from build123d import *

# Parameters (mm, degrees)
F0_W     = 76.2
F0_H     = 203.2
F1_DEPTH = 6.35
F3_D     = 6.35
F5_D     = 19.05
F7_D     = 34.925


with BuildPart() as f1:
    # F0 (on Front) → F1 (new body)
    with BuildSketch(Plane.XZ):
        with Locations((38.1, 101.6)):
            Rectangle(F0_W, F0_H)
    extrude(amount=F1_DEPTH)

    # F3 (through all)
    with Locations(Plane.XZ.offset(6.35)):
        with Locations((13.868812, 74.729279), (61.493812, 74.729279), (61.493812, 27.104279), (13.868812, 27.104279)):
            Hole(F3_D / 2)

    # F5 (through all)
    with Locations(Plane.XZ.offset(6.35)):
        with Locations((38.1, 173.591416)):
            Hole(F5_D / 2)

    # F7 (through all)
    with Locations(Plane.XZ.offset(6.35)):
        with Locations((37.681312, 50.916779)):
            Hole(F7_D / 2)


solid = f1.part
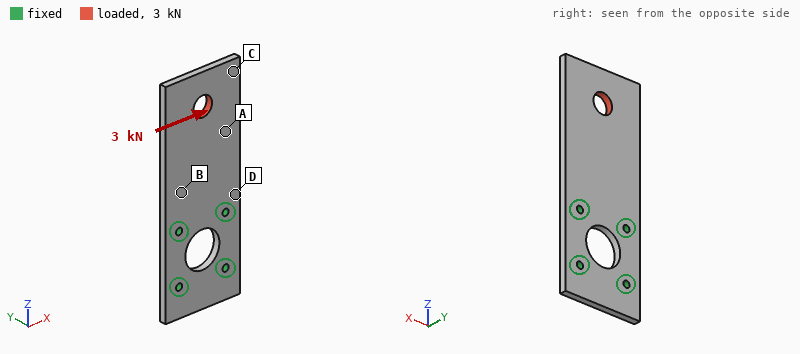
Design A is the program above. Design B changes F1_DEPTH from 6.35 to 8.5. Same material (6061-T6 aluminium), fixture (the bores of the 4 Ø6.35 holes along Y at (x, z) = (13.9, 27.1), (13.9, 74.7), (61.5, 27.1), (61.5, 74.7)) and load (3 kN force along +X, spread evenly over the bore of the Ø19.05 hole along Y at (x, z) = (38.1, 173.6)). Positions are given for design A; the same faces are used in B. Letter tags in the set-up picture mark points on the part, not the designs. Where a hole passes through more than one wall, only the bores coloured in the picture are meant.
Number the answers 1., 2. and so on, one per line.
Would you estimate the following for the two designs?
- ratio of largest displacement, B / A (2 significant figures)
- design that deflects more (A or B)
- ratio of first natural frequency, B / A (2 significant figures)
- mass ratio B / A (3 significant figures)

1. 0.75
2. A
3. 1.3
4. 1.34
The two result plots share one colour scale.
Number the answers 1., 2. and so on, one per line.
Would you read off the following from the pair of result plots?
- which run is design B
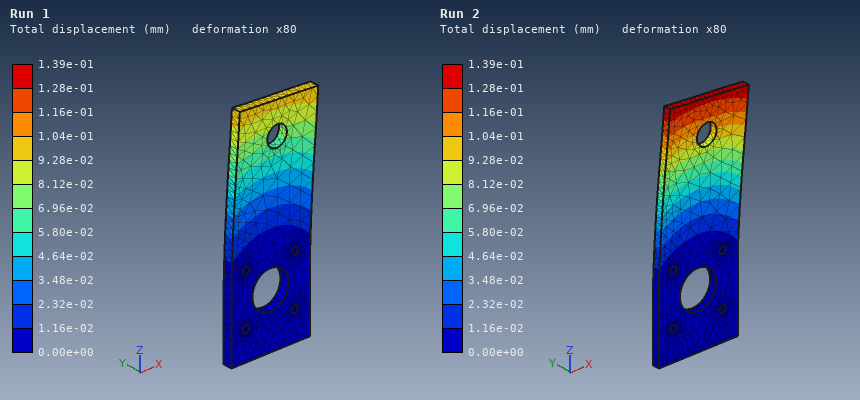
1. Run 1
